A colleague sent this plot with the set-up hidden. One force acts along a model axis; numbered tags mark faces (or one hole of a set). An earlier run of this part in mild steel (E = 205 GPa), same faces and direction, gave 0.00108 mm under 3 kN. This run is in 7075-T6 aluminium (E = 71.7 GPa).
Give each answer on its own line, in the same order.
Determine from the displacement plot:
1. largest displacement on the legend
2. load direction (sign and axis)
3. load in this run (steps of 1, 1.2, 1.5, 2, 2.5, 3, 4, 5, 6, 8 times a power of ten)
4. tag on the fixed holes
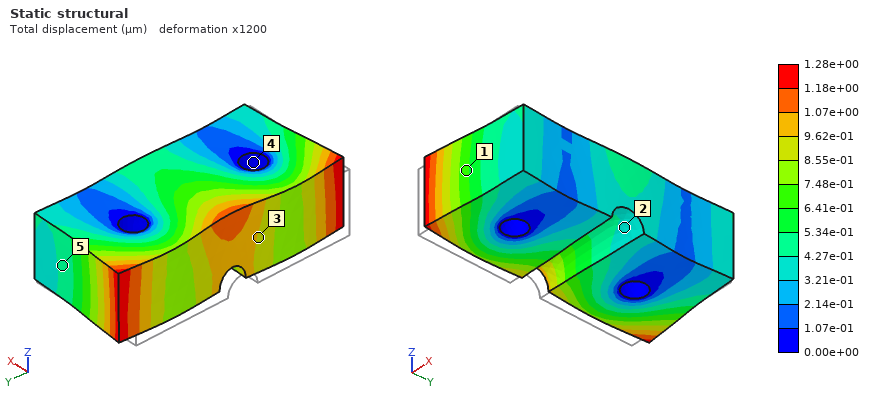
1.28e+00 µm
+X
1.2 kN
4
